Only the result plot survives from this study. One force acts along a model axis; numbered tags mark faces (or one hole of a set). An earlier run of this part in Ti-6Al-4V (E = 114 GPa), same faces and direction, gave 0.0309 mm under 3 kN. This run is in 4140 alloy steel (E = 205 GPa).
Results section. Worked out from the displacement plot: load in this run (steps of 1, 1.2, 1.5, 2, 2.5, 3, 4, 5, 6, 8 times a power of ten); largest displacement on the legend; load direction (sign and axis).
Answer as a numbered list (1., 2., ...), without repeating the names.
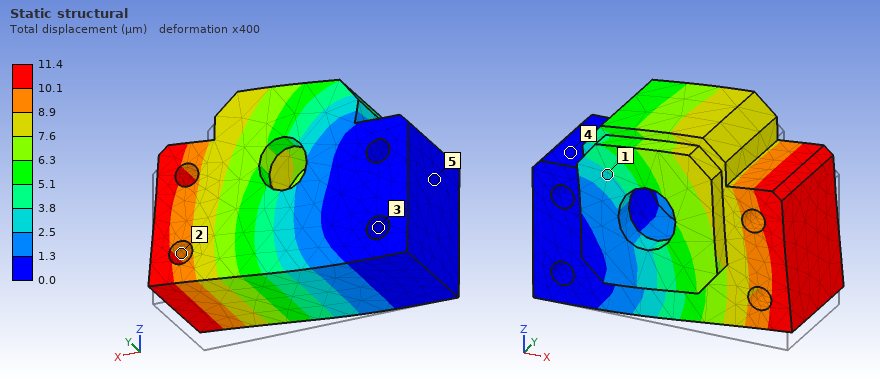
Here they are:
1. 2 kN
2. 11.4 µm
3. +Z
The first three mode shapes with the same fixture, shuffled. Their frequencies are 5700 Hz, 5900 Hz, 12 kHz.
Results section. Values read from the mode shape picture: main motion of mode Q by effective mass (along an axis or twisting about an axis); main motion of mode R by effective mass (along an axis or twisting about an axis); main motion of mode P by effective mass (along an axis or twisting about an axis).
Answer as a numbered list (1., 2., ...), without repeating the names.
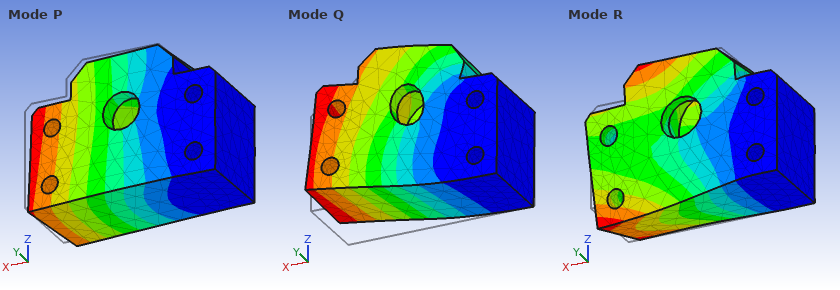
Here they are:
1. along Z
2. twisting about X
3. along Y
